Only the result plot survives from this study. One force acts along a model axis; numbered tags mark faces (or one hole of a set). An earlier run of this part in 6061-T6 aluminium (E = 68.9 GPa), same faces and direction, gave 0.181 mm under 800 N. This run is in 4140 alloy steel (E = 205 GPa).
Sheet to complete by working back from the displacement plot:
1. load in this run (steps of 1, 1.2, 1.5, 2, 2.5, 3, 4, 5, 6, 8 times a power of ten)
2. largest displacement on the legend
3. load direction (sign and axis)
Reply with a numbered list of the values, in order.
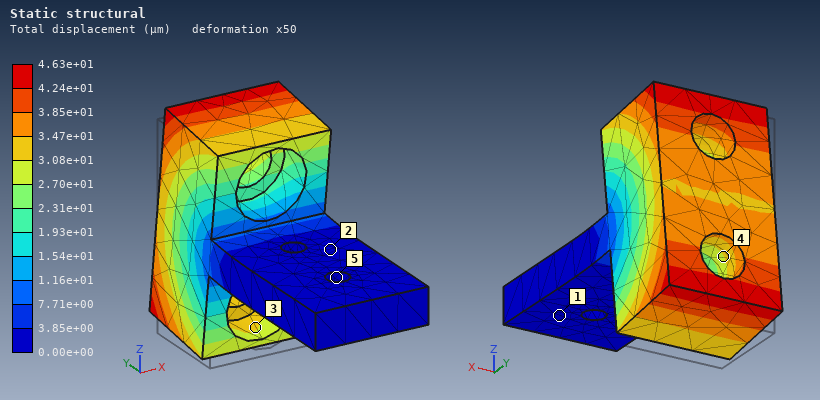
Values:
1. 600 N
2. 4.63e+01 µm
3. +Z
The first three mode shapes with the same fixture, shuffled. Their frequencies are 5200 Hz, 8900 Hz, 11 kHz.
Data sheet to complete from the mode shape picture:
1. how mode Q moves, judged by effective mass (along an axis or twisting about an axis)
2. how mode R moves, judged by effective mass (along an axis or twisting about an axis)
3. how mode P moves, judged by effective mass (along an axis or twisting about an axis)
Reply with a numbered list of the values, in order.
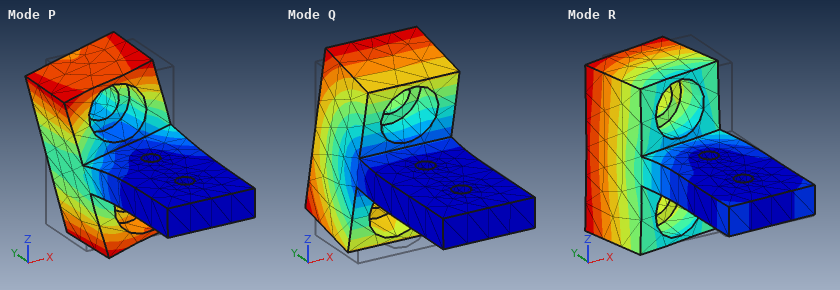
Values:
1. along Z
2. along X
3. twisting about Y
